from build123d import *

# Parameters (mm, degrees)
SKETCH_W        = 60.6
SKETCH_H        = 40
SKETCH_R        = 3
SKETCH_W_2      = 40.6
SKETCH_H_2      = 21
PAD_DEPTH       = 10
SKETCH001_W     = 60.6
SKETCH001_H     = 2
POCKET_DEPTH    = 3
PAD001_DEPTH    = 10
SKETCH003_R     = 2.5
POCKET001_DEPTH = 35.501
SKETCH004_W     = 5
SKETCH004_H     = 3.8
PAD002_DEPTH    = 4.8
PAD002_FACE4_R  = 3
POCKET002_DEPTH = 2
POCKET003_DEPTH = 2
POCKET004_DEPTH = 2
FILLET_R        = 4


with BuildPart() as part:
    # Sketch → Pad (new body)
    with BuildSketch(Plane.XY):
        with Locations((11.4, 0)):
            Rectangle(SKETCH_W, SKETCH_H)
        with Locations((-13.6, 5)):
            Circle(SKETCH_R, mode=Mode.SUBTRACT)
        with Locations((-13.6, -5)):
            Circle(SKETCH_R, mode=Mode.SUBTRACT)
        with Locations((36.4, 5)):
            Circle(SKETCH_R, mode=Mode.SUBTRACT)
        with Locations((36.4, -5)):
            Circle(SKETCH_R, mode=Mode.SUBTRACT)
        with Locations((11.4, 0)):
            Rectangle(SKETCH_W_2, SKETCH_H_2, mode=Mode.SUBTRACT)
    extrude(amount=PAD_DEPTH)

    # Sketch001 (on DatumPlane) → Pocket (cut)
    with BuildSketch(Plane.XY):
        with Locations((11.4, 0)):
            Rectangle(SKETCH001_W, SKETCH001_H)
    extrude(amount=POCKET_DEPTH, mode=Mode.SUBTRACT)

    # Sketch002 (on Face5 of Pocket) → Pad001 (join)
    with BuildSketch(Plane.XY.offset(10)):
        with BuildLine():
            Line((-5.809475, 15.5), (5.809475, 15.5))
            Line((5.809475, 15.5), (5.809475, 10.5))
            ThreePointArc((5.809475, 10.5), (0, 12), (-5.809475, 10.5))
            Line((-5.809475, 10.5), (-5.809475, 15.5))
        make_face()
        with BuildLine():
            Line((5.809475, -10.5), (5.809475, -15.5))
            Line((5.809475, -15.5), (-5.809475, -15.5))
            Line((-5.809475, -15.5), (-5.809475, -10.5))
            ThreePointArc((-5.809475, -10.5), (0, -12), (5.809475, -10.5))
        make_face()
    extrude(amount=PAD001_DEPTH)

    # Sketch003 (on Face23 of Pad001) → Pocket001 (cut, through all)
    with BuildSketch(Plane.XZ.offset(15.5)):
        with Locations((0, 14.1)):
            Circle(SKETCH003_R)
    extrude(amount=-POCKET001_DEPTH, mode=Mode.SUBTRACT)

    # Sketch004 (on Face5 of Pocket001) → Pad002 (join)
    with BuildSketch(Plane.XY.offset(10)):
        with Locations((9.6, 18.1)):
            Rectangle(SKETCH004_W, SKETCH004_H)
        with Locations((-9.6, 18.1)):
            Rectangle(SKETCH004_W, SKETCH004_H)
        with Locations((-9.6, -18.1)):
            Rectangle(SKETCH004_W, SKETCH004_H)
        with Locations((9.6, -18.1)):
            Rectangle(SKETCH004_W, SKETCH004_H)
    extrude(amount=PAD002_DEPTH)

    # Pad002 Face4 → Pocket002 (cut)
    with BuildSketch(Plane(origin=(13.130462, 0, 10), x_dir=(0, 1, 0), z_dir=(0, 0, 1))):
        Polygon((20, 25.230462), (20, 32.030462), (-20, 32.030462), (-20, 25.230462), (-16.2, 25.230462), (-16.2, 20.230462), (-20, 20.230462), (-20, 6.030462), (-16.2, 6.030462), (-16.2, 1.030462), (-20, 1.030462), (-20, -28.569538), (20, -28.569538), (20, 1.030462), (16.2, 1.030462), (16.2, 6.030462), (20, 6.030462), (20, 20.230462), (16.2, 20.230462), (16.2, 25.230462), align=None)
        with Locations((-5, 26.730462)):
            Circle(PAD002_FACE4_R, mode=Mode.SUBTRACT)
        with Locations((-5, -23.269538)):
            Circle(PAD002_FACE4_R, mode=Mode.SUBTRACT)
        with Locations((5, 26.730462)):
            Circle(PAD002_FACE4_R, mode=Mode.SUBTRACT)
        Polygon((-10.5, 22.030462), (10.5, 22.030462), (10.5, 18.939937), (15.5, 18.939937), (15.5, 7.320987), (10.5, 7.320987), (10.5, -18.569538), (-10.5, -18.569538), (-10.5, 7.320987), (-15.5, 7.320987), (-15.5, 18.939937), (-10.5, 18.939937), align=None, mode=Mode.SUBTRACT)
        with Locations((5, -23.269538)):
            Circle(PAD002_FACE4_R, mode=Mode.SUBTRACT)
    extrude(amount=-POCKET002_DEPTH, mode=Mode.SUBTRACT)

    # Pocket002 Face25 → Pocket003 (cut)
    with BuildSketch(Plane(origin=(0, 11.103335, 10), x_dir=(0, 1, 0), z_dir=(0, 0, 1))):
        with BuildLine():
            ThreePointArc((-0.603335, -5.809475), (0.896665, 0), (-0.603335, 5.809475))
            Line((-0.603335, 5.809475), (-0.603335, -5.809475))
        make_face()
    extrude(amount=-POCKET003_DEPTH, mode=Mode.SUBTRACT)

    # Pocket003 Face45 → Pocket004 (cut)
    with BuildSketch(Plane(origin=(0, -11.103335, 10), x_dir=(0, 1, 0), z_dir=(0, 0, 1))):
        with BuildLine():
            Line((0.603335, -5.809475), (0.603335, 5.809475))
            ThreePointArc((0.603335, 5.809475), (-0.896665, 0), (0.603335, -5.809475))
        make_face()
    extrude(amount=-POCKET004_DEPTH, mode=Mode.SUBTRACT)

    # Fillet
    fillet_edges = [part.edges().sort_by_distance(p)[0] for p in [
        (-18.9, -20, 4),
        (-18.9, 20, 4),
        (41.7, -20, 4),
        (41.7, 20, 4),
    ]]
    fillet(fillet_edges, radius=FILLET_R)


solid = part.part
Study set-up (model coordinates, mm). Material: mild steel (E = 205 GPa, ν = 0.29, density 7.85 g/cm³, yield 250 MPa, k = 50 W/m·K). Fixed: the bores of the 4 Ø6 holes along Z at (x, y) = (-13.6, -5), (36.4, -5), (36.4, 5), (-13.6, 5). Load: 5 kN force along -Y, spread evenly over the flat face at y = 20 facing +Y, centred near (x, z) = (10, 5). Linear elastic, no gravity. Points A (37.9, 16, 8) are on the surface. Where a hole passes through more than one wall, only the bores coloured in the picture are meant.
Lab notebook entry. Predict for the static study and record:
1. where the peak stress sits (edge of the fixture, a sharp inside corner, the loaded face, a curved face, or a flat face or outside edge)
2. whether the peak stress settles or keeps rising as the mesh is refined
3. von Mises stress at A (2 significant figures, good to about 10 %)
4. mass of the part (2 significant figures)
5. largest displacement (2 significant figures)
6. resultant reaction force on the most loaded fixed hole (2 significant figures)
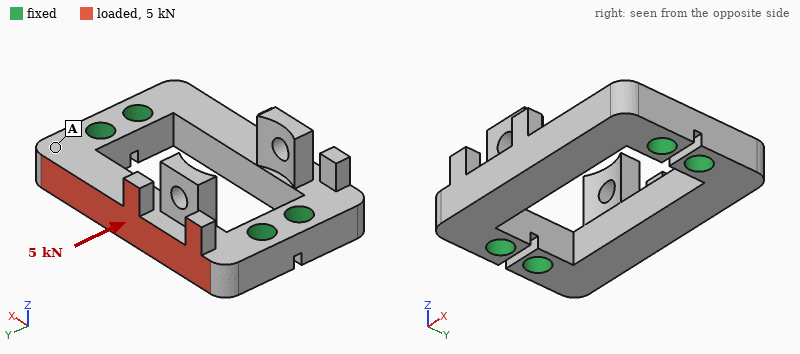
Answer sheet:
a sharp inside corner
keeps rising
21 MPa
100 g
36 µm
3.1 kN
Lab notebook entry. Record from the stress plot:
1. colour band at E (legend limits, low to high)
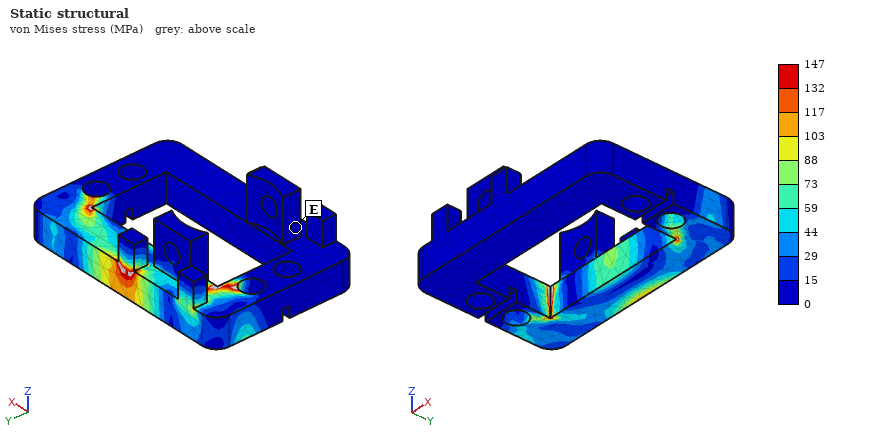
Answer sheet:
0 to 15 MPa
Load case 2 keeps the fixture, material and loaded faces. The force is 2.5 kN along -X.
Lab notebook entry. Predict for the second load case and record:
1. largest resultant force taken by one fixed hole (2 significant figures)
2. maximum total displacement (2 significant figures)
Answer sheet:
1.4 kN
8.0 µm
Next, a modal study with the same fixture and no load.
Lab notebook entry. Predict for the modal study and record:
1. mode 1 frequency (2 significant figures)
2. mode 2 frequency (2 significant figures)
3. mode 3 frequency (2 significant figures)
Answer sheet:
9600 Hz
9600 Hz
12 kHz
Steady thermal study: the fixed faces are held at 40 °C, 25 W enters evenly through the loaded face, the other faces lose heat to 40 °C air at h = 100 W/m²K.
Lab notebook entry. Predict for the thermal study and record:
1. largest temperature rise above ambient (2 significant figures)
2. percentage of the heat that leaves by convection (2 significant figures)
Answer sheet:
48 K
25 %
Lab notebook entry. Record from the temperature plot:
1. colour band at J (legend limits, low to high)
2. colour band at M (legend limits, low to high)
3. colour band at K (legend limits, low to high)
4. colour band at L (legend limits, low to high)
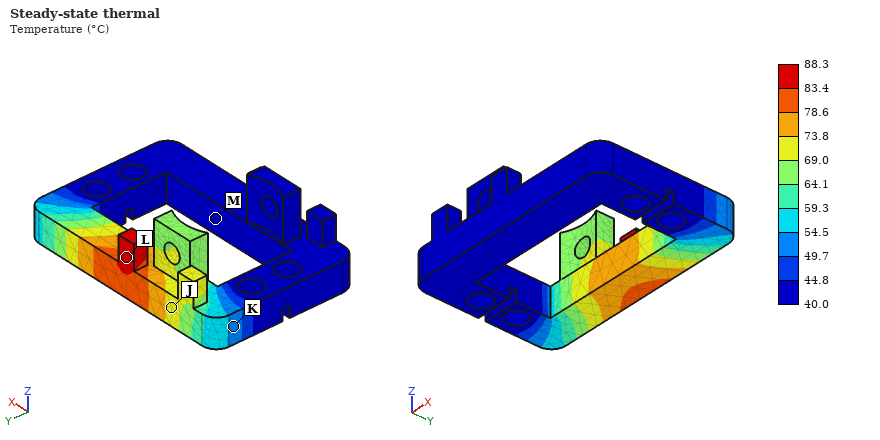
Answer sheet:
69.0 to 73.8 °C
40.0 to 44.8 °C
49.7 to 54.5 °C
83.4 to 88.3 °C
